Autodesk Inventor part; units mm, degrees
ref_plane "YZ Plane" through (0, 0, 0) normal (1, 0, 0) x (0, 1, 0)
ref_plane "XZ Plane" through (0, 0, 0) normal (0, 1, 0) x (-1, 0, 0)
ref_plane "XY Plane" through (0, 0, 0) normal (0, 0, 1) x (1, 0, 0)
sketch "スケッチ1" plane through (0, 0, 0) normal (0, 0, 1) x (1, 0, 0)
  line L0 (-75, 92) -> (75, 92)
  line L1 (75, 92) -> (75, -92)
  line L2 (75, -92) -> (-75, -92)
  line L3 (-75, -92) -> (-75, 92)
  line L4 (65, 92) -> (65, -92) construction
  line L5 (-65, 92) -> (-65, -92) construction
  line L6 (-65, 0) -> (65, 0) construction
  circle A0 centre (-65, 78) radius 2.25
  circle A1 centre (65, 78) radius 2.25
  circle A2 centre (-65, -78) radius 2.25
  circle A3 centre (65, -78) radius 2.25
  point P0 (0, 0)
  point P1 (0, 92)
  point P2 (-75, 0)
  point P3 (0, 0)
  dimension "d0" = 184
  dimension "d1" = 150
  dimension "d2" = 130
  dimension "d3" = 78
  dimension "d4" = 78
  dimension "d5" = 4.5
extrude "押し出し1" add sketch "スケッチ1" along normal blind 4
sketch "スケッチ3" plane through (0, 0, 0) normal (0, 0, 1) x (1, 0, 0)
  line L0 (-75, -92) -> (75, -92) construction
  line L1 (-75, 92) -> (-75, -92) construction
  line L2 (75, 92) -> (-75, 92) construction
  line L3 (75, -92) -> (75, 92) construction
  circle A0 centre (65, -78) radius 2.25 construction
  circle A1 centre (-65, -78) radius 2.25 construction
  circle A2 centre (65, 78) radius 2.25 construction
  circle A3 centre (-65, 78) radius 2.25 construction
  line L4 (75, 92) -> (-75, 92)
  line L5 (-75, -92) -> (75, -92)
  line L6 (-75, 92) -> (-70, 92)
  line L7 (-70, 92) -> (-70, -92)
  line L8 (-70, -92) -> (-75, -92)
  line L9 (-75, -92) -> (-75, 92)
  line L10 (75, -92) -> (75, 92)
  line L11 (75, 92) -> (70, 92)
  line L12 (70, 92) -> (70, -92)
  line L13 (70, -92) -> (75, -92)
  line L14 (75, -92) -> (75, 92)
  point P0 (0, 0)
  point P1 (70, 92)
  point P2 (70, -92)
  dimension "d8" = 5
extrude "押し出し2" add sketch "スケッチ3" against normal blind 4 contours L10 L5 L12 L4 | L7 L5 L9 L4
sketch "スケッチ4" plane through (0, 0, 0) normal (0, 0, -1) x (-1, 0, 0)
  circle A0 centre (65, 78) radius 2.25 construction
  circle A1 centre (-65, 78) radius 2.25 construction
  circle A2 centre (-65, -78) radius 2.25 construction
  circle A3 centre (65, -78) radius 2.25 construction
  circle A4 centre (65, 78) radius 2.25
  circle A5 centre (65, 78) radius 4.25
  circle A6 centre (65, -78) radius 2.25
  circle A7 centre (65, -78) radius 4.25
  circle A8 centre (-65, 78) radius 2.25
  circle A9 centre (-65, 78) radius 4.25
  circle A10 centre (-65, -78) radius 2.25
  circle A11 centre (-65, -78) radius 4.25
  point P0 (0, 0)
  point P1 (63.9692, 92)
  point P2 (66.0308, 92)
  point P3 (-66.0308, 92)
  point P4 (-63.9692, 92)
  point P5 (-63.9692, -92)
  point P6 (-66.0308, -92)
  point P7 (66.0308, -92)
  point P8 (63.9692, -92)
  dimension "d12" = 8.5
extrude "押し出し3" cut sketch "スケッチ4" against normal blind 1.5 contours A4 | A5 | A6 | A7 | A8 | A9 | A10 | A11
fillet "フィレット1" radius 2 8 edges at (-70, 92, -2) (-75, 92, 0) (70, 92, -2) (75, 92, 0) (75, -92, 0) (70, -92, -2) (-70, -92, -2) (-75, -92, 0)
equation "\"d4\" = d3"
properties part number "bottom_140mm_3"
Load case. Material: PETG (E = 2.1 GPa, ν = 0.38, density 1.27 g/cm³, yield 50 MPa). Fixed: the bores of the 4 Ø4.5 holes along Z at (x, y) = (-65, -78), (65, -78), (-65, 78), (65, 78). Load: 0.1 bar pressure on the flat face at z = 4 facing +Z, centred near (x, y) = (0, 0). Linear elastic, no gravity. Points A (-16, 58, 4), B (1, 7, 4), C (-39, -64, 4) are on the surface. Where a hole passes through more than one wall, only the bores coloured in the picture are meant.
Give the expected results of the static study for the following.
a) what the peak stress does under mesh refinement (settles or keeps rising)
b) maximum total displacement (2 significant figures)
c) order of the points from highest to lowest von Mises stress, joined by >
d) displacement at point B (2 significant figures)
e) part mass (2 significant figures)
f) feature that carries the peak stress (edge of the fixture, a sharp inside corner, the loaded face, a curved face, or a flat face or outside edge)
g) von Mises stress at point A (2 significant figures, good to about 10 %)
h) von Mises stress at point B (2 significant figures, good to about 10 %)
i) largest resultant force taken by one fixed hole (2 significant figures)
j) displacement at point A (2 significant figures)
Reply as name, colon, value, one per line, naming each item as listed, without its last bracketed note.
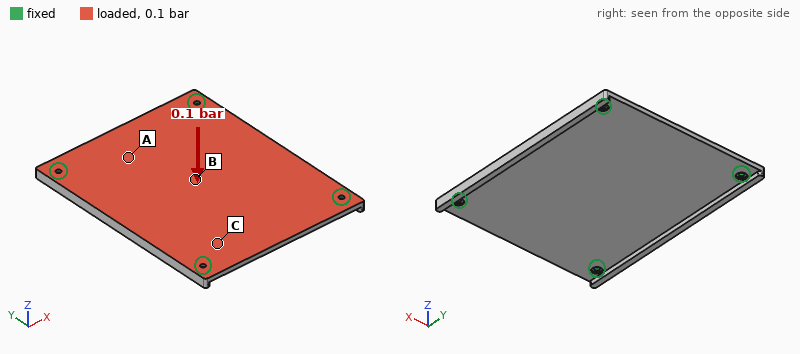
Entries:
what the peak stress does under mesh refinement: keeps rising
maximum total displacement: 2.7 mm
order of the points from highest to lowest von Mises stress, joined by >: B > A > C
displacement at point B: 2.7 mm
part mass: 150 g
feature that carries the peak stress: edge of the fixture
von Mises stress at point A: 3.3 MPa
von Mises stress at point B: 4.6 MPa
largest resultant force taken by one fixed hole: 130 N
displacement at point A: 1.7 mm
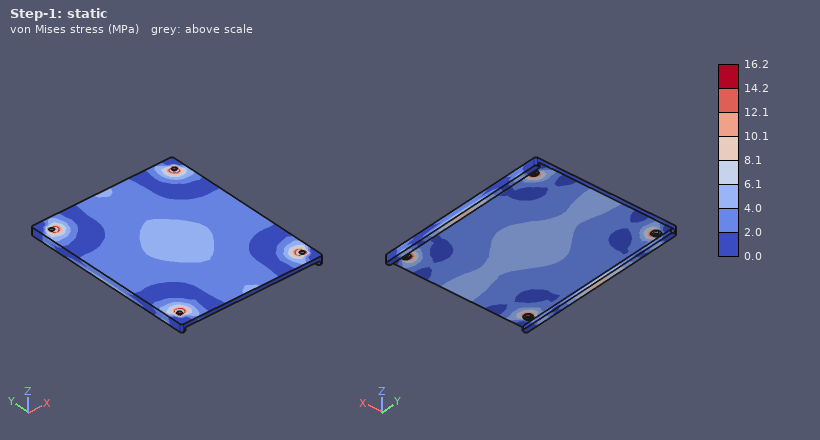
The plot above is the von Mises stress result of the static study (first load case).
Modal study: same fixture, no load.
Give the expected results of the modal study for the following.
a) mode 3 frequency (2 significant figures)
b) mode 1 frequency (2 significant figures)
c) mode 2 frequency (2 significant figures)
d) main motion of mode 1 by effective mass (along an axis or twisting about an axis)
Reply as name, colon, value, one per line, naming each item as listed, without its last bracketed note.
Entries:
mode 3 frequency: 290 Hz
mode 1 frequency: 160 Hz
mode 2 frequency: 280 Hz
main motion of mode 1 by effective mass: along Z
